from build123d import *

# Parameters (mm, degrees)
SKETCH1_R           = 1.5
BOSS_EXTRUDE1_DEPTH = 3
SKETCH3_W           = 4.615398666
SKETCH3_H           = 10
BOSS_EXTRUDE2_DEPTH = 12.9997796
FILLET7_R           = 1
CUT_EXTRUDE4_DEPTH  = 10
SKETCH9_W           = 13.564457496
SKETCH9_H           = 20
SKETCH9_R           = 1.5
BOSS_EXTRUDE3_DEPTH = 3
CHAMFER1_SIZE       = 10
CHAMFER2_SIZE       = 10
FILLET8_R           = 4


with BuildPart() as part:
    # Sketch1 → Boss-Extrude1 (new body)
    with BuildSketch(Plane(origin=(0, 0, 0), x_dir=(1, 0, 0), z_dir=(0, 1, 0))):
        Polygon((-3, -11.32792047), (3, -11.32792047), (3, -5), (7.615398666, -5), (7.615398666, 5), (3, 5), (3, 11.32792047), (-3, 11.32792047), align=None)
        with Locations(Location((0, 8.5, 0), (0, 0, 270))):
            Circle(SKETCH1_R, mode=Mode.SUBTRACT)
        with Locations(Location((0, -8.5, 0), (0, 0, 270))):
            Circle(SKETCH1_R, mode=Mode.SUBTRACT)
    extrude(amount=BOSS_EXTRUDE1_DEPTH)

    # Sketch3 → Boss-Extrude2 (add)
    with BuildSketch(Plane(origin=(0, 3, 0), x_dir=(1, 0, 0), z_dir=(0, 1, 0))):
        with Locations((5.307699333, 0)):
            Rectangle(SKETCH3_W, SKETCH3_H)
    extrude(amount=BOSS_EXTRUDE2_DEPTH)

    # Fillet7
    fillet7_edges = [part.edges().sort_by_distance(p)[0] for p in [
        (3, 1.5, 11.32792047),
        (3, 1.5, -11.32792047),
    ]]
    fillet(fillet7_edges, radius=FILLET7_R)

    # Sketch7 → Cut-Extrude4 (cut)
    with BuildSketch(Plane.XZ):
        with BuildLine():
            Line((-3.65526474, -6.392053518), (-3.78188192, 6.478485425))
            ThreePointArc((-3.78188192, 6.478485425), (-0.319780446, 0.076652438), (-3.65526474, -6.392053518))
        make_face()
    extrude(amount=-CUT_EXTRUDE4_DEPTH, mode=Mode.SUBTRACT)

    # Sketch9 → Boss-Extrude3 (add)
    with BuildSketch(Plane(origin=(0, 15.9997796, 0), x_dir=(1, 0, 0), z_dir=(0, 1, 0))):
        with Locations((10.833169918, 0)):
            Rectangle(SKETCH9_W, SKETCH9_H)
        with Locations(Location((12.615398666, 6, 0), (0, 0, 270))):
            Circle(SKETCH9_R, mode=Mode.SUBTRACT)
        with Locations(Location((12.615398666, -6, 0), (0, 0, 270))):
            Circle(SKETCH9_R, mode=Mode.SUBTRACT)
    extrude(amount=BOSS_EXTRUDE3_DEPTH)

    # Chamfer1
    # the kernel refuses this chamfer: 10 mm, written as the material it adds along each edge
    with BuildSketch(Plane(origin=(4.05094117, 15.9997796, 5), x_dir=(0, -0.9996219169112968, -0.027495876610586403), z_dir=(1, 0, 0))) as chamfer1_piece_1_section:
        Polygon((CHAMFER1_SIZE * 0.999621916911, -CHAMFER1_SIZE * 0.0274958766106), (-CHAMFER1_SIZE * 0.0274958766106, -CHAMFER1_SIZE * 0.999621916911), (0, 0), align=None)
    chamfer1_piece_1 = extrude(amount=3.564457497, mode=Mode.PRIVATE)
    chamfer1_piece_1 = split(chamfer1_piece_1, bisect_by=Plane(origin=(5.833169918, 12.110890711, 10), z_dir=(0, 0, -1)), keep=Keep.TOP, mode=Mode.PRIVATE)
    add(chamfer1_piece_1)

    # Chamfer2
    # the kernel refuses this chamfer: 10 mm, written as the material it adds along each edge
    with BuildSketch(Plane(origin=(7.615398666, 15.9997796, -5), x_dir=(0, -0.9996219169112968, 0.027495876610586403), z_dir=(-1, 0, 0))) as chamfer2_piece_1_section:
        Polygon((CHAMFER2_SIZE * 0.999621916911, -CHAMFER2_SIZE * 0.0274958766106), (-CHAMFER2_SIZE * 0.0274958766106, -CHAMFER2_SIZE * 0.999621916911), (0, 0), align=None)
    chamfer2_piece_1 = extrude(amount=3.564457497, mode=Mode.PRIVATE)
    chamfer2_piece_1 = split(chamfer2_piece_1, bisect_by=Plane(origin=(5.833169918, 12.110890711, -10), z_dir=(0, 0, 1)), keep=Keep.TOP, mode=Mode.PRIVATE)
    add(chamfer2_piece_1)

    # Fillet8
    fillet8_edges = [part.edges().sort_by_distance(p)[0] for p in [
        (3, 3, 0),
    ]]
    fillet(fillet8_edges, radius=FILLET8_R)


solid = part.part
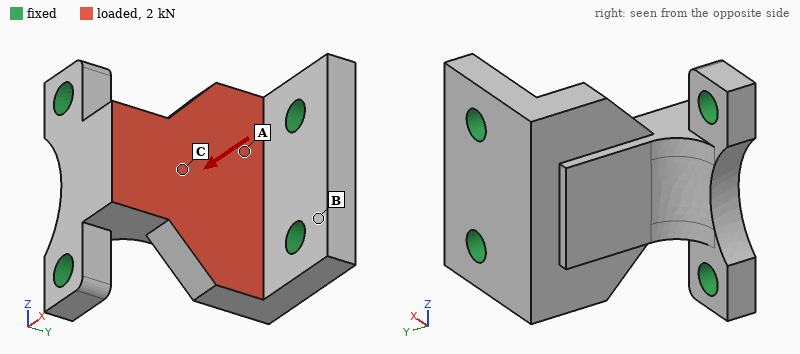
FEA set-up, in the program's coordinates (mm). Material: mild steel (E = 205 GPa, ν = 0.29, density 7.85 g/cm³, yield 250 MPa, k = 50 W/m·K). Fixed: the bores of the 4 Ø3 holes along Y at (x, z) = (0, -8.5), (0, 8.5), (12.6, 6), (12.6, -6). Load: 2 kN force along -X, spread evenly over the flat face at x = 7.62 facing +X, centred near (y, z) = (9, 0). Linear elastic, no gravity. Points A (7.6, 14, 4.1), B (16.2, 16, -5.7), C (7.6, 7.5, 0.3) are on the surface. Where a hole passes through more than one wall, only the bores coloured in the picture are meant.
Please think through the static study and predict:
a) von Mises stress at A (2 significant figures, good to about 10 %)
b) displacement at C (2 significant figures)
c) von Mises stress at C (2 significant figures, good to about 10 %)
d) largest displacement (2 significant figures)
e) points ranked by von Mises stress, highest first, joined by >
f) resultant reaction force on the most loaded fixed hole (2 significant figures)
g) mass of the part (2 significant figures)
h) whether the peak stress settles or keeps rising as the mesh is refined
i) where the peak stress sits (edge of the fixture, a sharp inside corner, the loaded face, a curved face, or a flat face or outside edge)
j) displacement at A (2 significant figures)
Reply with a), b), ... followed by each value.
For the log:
a) 32 MPa
b) 6.7 µm
c) 63 MPa
d) 8.5 µm
e) C > A > B
f) 550 N
g) 17 g
h) keeps rising
i) edge of the fixture
j) 4.0 µm
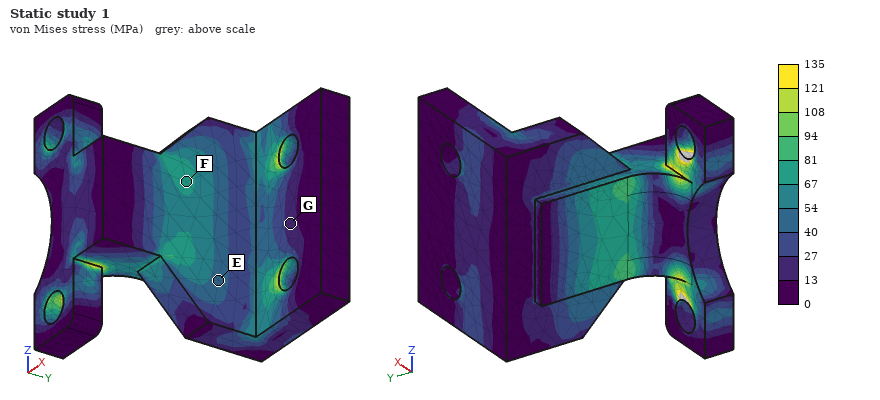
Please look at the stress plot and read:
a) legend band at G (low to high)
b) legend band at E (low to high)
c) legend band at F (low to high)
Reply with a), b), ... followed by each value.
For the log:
a) 13 to 27 MPa
b) 40 to 54 MPa
c) 67 to 81 MPa
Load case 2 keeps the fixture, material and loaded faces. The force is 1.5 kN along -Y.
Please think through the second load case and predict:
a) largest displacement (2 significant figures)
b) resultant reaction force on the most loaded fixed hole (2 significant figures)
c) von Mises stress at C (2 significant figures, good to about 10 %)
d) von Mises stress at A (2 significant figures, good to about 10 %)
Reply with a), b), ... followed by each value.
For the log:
a) 7.2 µm
b) 450 N
c) 47 MPa
d) 51 MPa
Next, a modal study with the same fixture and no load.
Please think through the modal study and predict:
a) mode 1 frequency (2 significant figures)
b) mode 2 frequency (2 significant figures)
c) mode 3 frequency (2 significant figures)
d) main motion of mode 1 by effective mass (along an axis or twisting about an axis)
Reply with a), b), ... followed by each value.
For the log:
a) 23 kHz
b) 42 kHz
c) 44 kHz
d) along Y
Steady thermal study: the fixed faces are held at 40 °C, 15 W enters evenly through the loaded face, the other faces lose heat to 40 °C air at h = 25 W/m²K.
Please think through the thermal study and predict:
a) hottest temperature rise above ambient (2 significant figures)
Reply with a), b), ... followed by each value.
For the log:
a) 30 K
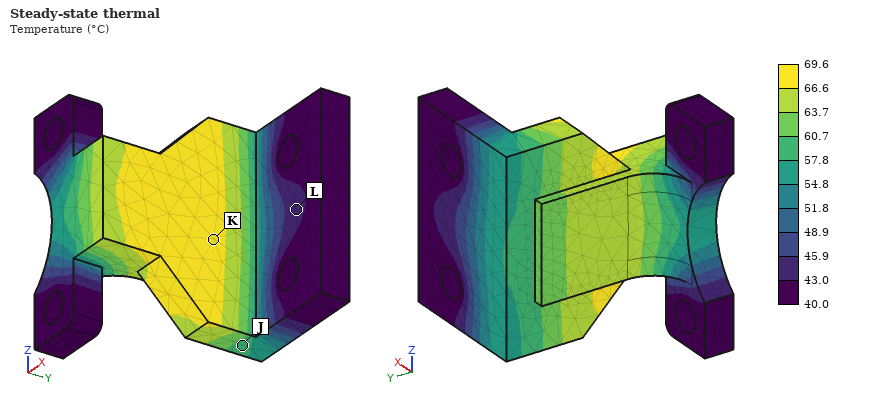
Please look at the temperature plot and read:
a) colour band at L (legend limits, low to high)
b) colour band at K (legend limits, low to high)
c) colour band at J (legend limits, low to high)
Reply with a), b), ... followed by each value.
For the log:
a) 43.0 to 45.9 °C
b) 66.6 to 69.6 °C
c) 57.8 to 60.7 °C
